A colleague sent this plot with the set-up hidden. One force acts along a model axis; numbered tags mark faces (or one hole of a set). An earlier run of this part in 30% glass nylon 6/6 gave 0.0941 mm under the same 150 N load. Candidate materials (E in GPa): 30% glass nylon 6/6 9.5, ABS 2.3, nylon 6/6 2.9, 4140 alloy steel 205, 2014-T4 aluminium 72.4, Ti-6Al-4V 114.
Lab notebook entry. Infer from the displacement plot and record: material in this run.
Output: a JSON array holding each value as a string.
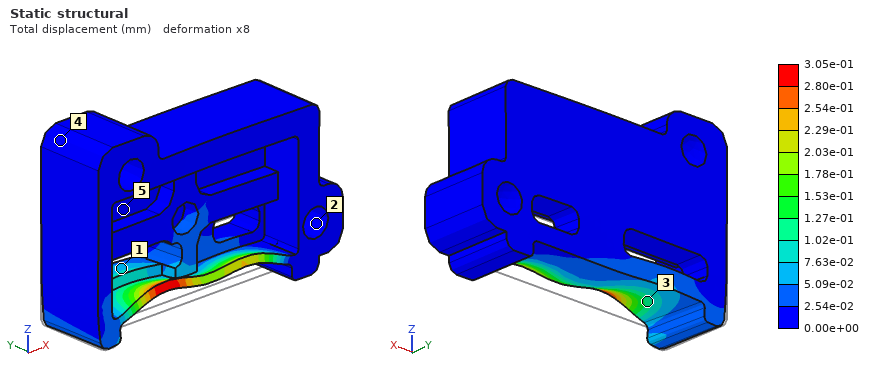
["nylon 6/6"]
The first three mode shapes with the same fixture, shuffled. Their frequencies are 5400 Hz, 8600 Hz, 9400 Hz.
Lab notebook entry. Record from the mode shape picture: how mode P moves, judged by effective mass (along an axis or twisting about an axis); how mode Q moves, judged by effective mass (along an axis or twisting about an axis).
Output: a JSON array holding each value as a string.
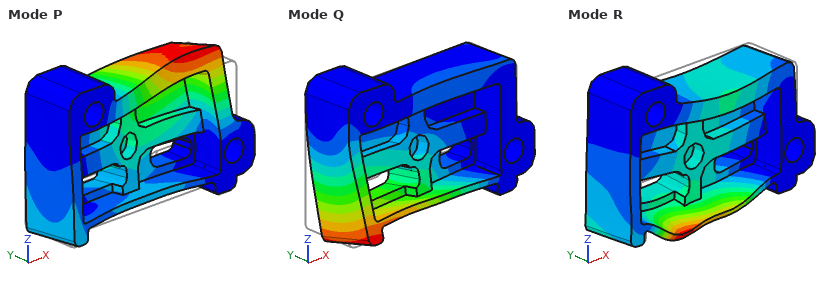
["along Y", "along Y"]
